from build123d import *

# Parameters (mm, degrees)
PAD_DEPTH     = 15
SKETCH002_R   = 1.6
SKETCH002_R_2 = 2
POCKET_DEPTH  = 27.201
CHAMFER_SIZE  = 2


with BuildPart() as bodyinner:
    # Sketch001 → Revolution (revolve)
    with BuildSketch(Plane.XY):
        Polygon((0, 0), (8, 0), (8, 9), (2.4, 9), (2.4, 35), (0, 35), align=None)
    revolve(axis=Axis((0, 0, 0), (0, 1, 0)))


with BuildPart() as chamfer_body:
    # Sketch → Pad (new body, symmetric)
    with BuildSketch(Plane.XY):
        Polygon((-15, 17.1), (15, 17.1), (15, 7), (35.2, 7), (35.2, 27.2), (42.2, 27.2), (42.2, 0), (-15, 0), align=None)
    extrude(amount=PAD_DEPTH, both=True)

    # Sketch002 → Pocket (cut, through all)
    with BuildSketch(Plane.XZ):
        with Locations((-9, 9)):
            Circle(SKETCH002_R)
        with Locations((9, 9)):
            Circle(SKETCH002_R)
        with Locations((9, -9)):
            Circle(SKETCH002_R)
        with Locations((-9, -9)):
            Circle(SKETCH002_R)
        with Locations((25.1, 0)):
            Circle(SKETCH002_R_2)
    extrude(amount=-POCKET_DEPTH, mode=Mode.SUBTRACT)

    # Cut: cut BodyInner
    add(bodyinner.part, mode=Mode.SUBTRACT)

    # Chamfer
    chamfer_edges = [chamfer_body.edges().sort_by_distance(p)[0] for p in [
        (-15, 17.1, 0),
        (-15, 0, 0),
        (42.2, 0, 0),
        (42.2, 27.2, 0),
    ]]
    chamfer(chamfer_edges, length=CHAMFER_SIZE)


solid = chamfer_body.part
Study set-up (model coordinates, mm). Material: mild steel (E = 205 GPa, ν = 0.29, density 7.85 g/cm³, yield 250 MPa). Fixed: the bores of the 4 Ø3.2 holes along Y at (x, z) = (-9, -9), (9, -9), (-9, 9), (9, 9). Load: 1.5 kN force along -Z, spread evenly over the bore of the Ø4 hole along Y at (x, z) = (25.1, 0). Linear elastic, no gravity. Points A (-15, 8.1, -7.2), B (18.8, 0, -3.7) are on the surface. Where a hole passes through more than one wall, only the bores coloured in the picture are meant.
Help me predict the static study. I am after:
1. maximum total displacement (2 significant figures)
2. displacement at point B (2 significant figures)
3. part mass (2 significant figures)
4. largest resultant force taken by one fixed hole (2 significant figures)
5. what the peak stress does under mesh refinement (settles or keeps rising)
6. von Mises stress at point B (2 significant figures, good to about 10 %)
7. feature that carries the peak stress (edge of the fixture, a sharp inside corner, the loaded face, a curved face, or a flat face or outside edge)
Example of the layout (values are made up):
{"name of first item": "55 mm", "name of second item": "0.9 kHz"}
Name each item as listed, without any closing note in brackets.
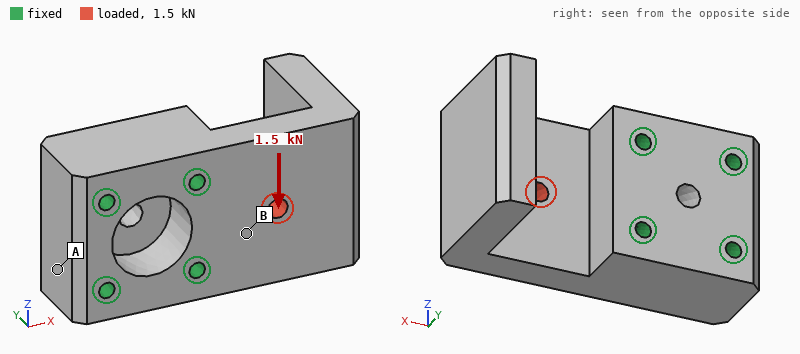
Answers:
{"maximum total displacement": "3.7 µm", "displacement at point B": "1.1 µm", "part mass": "180 g", "largest resultant force taken by one fixed hole": "1.3 kN", "what the peak stress does under mesh refinement": "keeps rising", "von Mises stress at point B": "16 MPa", "feature that carries the peak stress": "edge of the fixture"}
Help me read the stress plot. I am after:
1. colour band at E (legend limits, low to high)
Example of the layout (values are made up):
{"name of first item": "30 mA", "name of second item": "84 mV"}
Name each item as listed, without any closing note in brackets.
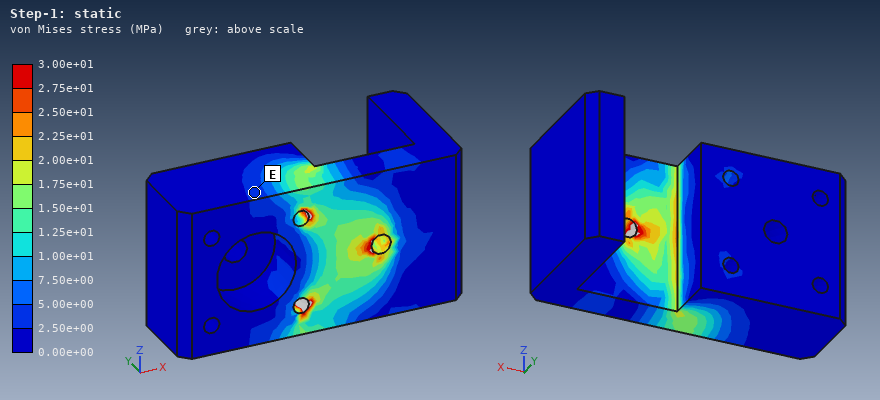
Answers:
{"colour band at E": "2.50e+00 to 5.00e+00 MPa"}
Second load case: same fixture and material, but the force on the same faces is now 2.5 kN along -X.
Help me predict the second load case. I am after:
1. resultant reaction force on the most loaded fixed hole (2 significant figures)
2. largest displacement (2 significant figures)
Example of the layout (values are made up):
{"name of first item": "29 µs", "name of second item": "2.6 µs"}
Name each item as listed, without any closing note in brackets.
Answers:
{"resultant reaction force on the most loaded fixed hole": "1.2 kN", "largest displacement": "2.1 µm"}
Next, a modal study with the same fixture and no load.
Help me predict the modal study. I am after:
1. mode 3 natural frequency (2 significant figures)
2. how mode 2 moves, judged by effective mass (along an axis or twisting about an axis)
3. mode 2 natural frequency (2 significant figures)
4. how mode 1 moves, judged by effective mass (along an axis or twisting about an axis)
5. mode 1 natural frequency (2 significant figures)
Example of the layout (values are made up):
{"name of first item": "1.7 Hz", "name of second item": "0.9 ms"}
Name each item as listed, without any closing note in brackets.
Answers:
{"mode 3 natural frequency": "8600 Hz", "how mode 2 moves, judged by effective mass": "along Z", "mode 2 natural frequency": "5100 Hz", "how mode 1 moves, judged by effective mass": "along Y", "mode 1 natural frequency": "2900 Hz"}
